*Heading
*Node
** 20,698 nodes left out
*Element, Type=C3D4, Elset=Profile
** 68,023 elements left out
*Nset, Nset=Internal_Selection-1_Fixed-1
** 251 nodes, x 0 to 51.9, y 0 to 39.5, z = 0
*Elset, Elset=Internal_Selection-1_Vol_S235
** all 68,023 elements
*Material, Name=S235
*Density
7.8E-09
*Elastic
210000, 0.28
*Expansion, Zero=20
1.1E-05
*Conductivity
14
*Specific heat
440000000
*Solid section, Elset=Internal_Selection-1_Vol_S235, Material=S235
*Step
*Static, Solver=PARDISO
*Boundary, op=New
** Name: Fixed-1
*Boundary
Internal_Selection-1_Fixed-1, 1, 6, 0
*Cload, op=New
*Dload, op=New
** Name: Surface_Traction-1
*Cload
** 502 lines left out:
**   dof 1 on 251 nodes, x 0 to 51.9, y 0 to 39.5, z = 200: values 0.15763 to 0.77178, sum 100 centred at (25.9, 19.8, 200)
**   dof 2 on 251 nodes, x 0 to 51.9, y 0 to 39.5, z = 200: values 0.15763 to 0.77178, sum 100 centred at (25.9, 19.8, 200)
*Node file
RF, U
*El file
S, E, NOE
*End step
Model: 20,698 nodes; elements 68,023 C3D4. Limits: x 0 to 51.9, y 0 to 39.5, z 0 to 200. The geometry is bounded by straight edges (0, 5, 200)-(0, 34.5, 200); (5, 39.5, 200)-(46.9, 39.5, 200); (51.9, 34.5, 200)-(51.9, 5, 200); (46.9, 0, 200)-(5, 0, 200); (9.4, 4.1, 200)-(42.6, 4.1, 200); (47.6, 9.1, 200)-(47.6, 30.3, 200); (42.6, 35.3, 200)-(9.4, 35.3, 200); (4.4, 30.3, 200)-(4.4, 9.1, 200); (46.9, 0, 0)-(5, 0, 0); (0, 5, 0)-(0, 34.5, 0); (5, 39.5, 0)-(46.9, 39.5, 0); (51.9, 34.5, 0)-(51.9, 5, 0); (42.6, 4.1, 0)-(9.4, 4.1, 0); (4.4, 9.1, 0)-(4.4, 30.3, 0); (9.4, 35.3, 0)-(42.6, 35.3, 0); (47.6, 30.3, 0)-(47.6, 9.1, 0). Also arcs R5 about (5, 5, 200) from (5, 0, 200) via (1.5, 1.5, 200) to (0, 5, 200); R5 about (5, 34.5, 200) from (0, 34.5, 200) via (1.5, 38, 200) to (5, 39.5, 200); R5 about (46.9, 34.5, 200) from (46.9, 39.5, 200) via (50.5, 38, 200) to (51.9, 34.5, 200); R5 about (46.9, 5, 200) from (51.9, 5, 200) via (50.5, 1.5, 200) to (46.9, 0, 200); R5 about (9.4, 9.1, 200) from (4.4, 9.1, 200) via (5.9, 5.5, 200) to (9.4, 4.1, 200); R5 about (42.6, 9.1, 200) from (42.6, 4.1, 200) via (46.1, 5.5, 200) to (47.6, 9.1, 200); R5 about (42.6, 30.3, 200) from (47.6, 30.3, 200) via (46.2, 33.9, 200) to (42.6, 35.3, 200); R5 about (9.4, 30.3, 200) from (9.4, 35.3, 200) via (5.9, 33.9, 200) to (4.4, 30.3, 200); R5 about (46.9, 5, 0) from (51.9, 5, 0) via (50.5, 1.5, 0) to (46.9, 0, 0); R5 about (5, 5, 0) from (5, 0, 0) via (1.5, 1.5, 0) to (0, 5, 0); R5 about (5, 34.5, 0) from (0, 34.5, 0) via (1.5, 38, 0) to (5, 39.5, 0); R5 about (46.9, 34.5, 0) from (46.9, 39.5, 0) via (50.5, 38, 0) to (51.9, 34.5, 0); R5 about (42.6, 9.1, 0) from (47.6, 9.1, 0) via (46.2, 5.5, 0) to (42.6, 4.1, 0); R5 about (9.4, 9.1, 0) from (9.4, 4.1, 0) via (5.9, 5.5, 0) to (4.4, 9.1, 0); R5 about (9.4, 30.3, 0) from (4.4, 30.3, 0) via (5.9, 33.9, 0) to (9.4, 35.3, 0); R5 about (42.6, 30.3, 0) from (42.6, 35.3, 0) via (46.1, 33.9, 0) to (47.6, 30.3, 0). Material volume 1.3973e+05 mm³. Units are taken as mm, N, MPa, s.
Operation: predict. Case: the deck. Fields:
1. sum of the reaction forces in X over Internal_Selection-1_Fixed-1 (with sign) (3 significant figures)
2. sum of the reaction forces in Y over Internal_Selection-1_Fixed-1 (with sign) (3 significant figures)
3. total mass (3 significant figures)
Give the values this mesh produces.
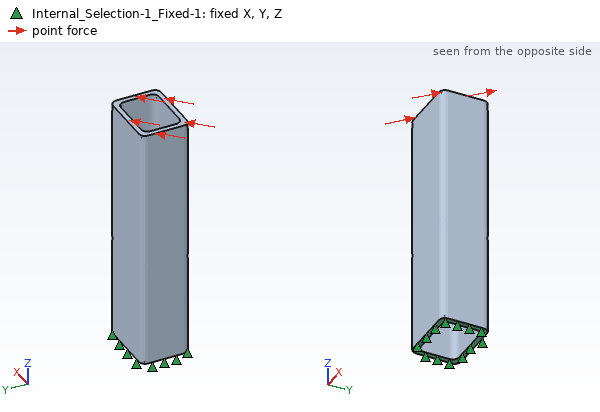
-100 N
-100 N
1.09 kg
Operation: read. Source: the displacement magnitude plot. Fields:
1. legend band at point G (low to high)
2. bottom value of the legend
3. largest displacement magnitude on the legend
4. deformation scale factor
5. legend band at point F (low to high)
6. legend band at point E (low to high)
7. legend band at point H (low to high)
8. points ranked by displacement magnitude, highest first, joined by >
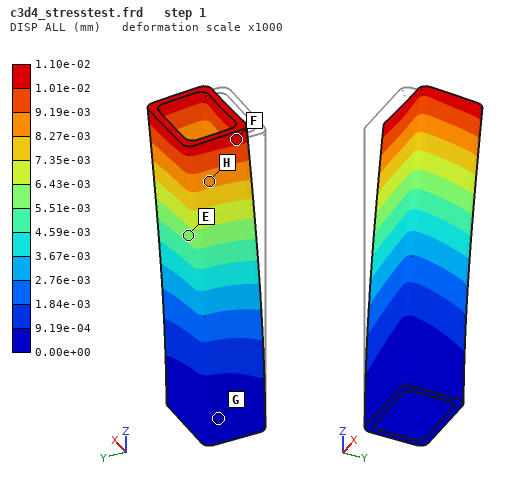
0.00e+00 to 9.19e-04 mm
0.00e+00 mm
1.10e-02 mm
1000
1.01e-02 to 1.10e-02 mm
5.51e-03 to 6.43e-03 mm
8.27e-03 to 9.19e-03 mm
F > H > E > G
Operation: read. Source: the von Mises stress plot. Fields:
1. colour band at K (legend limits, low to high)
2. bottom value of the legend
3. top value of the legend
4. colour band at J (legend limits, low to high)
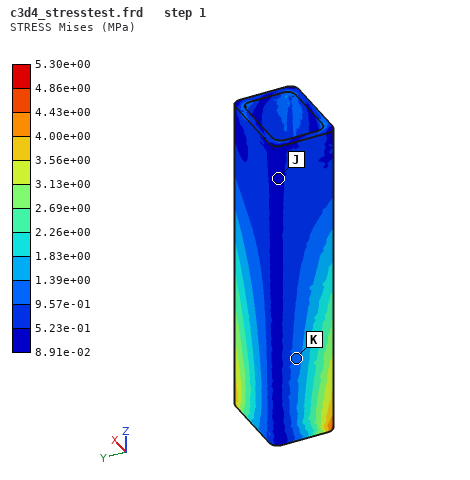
9.57e-01 to 1.39e+00 MPa
8.91e-02 MPa
5.30e+00 MPa
8.91e-02 to 5.23e-01 MPa
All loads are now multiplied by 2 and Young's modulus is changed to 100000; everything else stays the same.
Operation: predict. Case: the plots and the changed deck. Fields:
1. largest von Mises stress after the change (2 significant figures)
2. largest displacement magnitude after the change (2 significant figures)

11 MPa
0.046 mm
